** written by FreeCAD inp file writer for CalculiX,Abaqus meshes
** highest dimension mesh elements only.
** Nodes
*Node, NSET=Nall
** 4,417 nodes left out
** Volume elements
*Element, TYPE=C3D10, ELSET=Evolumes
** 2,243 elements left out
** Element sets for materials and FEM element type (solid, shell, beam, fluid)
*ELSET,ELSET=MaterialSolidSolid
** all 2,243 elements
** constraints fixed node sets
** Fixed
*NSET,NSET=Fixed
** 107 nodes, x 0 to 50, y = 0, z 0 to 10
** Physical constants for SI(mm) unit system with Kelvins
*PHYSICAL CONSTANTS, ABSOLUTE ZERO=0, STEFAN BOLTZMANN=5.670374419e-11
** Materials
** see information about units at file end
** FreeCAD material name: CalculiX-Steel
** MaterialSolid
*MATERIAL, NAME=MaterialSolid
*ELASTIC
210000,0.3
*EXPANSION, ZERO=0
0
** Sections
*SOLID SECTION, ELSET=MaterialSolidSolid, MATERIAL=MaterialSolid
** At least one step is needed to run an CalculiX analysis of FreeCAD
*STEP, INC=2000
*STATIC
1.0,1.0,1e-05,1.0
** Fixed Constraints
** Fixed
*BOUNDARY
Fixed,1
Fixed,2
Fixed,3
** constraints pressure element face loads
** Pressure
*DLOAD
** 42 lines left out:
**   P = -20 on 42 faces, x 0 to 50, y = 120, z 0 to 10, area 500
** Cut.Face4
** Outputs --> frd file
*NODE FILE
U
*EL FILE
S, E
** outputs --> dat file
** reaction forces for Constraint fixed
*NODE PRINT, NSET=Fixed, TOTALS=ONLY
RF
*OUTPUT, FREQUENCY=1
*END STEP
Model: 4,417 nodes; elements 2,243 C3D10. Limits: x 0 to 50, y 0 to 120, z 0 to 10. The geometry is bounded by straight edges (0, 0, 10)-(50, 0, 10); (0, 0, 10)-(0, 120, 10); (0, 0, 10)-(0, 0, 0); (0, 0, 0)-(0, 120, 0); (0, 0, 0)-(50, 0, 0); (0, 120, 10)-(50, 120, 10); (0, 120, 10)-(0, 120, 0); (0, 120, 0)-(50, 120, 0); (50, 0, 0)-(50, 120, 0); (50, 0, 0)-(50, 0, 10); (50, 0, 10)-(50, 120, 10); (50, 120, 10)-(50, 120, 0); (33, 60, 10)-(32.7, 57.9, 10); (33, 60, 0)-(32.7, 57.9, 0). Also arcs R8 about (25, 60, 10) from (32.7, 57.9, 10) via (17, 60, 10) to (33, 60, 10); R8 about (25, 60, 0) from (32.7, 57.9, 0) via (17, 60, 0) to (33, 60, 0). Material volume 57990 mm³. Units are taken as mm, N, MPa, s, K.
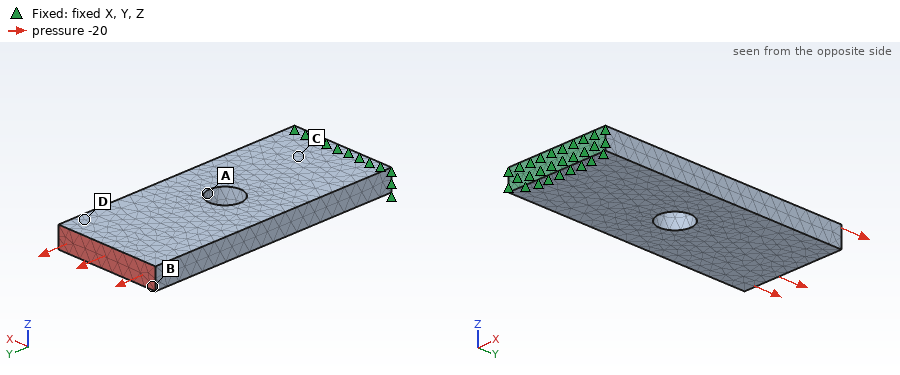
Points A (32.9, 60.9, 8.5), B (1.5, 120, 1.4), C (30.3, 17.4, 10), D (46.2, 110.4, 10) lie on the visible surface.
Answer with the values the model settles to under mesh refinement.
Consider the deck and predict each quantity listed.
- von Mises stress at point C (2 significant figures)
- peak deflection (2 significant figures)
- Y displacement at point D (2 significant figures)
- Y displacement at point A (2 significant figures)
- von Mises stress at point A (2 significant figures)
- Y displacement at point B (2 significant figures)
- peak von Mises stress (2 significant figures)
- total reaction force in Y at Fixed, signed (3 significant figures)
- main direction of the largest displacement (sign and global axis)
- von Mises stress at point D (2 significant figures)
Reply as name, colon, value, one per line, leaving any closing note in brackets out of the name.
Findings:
von Mises stress at point C: 19 MPa
peak deflection: 0.013 mm
Y displacement at point D: 0.012 mm
Y displacement at point A: 0.0066 mm
von Mises stress at point A: 67 MPa
Y displacement at point B: 0.013 mm
peak von Mises stress: 69 MPa
total reaction force in Y at Fixed, signed: -10000 N
main direction of the largest displacement: +Y
von Mises stress at point D: 20 MPa
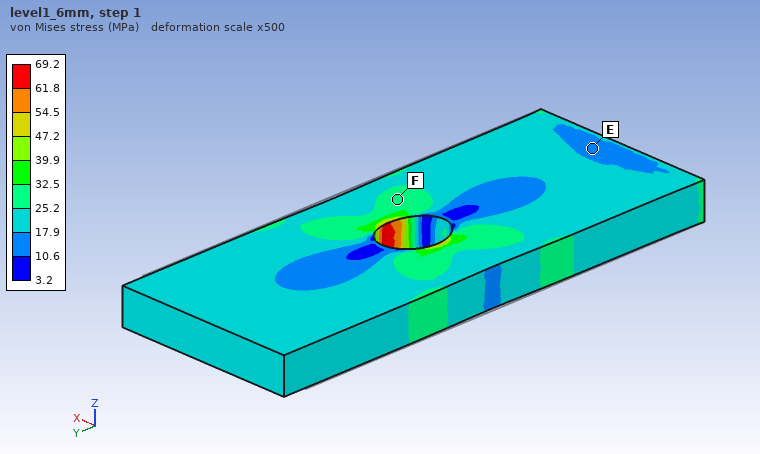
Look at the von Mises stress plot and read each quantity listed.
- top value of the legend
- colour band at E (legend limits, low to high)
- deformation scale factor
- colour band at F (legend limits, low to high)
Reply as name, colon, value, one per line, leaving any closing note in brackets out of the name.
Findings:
top value of the legend: 69.2 MPa
colour band at E: 10.6 to 17.9 MPa
deformation scale factor: 500
colour band at F: 25.2 to 32.5 MPa
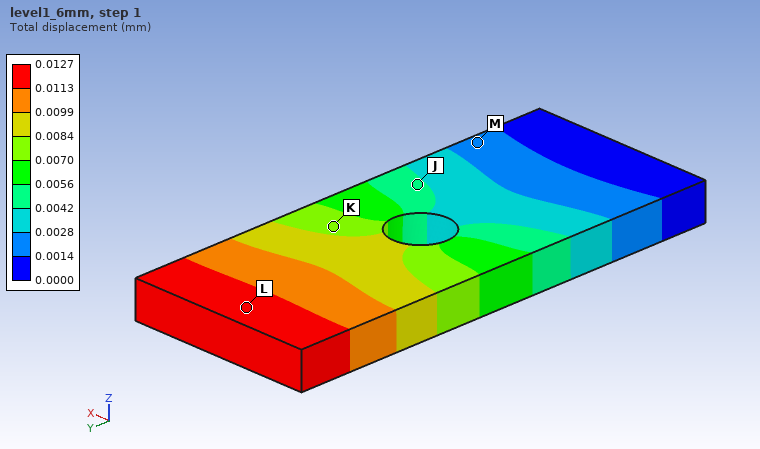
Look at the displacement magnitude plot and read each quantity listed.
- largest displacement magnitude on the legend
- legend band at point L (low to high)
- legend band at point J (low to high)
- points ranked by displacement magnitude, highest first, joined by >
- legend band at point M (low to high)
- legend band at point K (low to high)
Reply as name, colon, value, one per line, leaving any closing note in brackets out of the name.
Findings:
largest displacement magnitude on the legend: 0.0127 mm
legend band at point L: 0.0113 to 0.0127 mm
legend band at point J: 0.0042 to 0.0056 mm
points ranked by displacement magnitude, highest first, joined by >: L > K > J > M
legend band at point M: 0.0014 to 0.0028 mm
legend band at point K: 0.0070 to 0.0084 mm
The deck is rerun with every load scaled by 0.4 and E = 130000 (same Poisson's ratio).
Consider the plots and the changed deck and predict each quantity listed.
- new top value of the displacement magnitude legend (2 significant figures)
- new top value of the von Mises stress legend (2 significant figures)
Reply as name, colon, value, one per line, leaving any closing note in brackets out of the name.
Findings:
new top value of the displacement magnitude legend: 0.0082 mm
new top value of the von Mises stress legend: 28 MPa
